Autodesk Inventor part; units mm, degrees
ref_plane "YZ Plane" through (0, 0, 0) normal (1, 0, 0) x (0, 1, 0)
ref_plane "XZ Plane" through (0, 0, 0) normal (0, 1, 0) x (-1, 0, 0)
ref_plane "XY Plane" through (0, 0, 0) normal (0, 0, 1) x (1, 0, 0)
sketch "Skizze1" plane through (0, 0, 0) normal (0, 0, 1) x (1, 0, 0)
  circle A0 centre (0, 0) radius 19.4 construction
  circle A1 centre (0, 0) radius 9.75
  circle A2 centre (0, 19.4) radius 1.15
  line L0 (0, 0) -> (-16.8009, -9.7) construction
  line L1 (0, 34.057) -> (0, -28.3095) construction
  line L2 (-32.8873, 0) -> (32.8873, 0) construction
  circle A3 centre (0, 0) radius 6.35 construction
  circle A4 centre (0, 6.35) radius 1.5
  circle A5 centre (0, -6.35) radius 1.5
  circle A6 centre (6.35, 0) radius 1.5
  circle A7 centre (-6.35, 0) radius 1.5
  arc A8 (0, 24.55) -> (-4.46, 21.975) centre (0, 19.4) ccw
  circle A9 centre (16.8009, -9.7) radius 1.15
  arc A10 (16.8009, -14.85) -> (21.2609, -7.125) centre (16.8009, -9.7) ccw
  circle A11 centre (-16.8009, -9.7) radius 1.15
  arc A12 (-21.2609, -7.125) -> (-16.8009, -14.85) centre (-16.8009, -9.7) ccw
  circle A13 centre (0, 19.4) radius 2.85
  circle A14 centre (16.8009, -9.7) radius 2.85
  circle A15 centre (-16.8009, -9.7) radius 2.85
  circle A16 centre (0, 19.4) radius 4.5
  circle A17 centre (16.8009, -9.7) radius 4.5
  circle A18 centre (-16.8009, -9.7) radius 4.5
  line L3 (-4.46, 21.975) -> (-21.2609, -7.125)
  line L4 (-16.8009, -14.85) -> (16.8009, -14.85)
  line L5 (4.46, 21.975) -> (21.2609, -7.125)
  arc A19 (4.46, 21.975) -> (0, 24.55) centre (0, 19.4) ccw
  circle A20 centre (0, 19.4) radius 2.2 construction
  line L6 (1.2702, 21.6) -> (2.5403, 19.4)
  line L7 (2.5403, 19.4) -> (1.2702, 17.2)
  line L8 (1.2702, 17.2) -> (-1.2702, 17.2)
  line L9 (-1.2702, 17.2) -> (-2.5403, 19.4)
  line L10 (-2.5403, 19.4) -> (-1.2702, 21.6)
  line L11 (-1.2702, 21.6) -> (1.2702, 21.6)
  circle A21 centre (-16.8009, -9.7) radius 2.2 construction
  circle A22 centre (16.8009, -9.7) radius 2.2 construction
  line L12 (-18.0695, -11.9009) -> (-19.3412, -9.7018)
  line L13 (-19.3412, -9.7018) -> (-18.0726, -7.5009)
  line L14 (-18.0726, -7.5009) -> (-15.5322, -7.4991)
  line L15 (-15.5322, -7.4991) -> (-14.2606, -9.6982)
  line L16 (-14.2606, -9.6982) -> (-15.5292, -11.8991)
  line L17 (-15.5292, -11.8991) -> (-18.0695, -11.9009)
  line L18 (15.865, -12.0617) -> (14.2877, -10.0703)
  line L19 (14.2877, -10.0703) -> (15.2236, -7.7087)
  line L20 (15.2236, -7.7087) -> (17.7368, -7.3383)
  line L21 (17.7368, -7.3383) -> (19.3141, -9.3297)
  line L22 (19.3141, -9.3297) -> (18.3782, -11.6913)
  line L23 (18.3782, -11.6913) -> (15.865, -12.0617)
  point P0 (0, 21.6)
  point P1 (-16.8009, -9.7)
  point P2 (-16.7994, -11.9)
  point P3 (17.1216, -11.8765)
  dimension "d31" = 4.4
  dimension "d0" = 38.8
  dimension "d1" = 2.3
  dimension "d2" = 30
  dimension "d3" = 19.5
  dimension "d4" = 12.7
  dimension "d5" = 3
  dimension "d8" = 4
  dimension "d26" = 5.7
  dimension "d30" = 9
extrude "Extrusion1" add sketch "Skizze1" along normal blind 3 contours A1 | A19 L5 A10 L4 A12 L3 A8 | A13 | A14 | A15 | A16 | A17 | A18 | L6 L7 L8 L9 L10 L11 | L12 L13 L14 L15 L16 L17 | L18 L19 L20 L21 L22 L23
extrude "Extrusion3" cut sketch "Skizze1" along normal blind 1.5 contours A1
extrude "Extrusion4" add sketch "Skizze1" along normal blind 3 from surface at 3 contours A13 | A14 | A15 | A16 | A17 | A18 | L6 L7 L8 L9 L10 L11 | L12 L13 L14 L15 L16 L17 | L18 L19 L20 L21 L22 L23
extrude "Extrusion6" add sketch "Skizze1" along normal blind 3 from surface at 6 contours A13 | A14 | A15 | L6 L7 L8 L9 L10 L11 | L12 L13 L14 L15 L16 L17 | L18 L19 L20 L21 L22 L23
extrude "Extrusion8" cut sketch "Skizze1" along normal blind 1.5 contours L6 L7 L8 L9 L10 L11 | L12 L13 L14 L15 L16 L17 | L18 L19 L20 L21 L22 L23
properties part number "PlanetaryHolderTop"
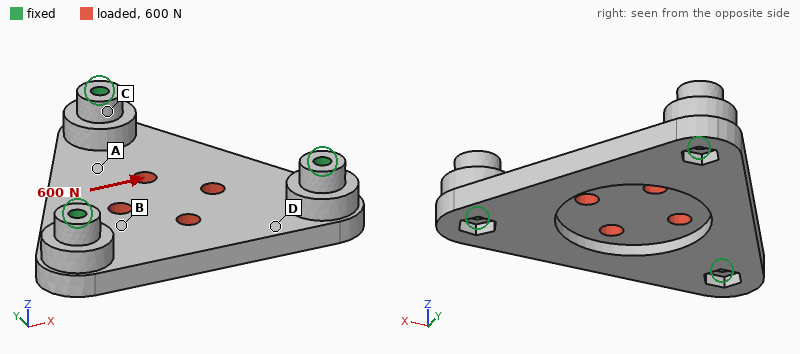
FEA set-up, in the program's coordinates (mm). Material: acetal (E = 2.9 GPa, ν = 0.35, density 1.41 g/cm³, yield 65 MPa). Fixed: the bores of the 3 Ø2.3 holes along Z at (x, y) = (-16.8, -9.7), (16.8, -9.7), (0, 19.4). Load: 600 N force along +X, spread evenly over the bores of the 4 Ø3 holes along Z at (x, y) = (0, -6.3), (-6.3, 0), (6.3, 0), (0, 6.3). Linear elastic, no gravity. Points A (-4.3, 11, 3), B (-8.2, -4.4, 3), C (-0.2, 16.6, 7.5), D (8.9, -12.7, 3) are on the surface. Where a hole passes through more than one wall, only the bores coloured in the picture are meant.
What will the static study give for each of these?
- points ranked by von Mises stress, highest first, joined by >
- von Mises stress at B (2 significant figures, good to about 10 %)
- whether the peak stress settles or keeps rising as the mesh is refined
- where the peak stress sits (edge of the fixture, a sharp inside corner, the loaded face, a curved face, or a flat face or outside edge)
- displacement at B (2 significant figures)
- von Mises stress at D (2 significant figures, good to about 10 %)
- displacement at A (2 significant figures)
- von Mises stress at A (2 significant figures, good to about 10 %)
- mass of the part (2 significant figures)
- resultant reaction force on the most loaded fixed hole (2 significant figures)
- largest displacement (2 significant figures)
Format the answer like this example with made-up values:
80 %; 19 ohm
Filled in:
B > D > A > C; 14 MPa; keeps rising; edge of the fixture; 50 µm; 8.2 MPa; 55 µm; 4.6 MPa; 4.8 g; 240 N; 93 µm
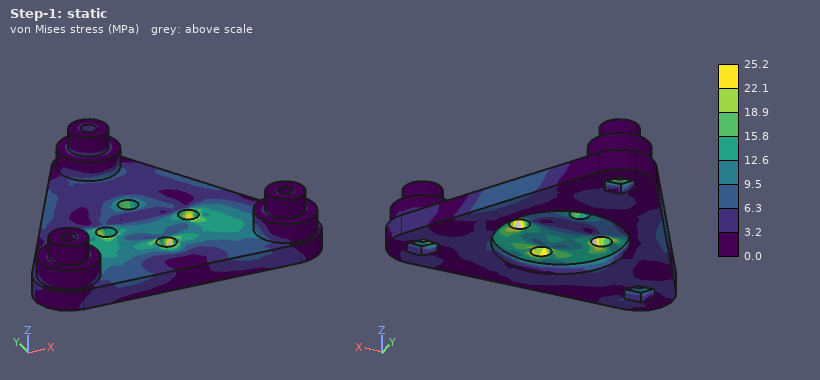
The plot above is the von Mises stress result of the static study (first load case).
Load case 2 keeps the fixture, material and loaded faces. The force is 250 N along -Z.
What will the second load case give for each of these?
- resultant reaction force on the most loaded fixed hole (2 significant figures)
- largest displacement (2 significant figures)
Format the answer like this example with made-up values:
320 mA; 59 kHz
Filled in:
89 N; 0.53 mm
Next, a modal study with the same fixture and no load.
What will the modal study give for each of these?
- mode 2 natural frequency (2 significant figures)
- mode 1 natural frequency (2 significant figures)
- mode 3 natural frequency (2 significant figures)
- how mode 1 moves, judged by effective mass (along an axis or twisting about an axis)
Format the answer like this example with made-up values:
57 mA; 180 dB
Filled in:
5100 Hz; 4200 Hz; 5100 Hz; along Z
